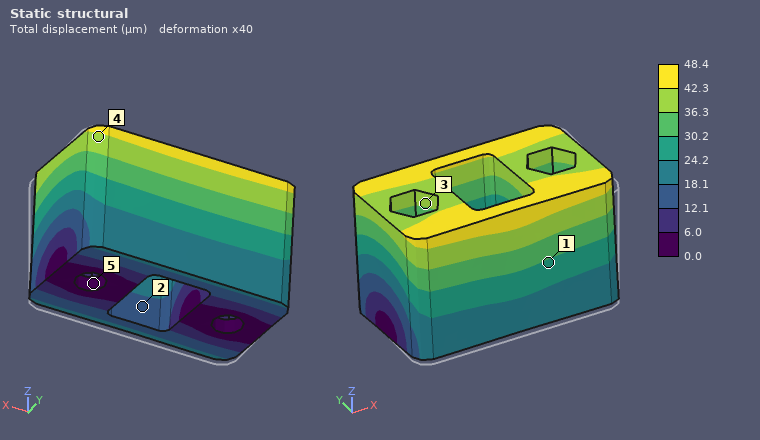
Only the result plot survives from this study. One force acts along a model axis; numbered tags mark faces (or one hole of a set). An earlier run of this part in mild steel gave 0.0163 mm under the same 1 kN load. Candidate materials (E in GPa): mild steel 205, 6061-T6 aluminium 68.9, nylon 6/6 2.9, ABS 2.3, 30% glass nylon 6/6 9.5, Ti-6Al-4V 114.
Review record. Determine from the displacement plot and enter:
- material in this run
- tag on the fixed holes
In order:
6061-T6 aluminium
5
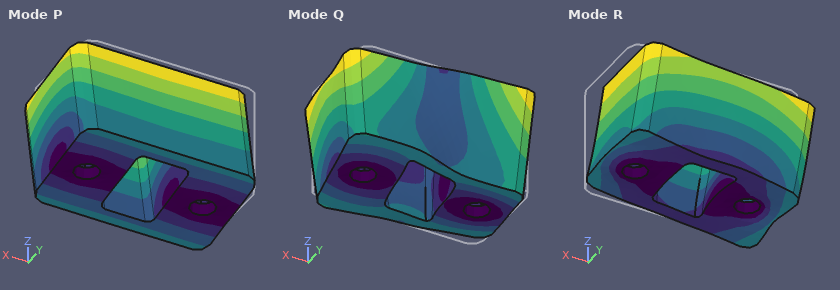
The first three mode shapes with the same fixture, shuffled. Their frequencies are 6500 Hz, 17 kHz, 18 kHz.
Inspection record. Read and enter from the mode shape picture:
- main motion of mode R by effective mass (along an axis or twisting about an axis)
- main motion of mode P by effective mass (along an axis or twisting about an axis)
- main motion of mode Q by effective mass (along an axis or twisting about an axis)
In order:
along X
along Y
twisting about Z
